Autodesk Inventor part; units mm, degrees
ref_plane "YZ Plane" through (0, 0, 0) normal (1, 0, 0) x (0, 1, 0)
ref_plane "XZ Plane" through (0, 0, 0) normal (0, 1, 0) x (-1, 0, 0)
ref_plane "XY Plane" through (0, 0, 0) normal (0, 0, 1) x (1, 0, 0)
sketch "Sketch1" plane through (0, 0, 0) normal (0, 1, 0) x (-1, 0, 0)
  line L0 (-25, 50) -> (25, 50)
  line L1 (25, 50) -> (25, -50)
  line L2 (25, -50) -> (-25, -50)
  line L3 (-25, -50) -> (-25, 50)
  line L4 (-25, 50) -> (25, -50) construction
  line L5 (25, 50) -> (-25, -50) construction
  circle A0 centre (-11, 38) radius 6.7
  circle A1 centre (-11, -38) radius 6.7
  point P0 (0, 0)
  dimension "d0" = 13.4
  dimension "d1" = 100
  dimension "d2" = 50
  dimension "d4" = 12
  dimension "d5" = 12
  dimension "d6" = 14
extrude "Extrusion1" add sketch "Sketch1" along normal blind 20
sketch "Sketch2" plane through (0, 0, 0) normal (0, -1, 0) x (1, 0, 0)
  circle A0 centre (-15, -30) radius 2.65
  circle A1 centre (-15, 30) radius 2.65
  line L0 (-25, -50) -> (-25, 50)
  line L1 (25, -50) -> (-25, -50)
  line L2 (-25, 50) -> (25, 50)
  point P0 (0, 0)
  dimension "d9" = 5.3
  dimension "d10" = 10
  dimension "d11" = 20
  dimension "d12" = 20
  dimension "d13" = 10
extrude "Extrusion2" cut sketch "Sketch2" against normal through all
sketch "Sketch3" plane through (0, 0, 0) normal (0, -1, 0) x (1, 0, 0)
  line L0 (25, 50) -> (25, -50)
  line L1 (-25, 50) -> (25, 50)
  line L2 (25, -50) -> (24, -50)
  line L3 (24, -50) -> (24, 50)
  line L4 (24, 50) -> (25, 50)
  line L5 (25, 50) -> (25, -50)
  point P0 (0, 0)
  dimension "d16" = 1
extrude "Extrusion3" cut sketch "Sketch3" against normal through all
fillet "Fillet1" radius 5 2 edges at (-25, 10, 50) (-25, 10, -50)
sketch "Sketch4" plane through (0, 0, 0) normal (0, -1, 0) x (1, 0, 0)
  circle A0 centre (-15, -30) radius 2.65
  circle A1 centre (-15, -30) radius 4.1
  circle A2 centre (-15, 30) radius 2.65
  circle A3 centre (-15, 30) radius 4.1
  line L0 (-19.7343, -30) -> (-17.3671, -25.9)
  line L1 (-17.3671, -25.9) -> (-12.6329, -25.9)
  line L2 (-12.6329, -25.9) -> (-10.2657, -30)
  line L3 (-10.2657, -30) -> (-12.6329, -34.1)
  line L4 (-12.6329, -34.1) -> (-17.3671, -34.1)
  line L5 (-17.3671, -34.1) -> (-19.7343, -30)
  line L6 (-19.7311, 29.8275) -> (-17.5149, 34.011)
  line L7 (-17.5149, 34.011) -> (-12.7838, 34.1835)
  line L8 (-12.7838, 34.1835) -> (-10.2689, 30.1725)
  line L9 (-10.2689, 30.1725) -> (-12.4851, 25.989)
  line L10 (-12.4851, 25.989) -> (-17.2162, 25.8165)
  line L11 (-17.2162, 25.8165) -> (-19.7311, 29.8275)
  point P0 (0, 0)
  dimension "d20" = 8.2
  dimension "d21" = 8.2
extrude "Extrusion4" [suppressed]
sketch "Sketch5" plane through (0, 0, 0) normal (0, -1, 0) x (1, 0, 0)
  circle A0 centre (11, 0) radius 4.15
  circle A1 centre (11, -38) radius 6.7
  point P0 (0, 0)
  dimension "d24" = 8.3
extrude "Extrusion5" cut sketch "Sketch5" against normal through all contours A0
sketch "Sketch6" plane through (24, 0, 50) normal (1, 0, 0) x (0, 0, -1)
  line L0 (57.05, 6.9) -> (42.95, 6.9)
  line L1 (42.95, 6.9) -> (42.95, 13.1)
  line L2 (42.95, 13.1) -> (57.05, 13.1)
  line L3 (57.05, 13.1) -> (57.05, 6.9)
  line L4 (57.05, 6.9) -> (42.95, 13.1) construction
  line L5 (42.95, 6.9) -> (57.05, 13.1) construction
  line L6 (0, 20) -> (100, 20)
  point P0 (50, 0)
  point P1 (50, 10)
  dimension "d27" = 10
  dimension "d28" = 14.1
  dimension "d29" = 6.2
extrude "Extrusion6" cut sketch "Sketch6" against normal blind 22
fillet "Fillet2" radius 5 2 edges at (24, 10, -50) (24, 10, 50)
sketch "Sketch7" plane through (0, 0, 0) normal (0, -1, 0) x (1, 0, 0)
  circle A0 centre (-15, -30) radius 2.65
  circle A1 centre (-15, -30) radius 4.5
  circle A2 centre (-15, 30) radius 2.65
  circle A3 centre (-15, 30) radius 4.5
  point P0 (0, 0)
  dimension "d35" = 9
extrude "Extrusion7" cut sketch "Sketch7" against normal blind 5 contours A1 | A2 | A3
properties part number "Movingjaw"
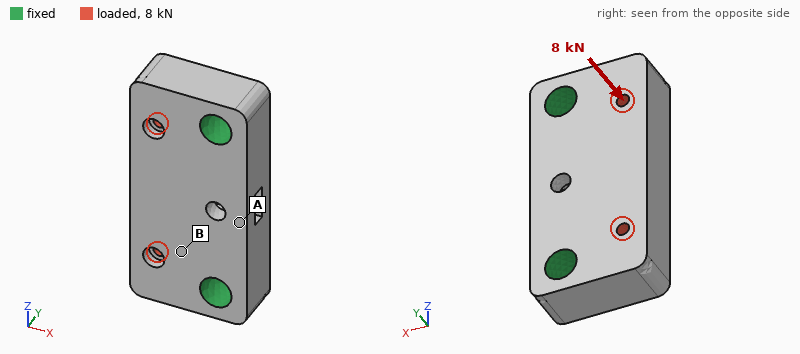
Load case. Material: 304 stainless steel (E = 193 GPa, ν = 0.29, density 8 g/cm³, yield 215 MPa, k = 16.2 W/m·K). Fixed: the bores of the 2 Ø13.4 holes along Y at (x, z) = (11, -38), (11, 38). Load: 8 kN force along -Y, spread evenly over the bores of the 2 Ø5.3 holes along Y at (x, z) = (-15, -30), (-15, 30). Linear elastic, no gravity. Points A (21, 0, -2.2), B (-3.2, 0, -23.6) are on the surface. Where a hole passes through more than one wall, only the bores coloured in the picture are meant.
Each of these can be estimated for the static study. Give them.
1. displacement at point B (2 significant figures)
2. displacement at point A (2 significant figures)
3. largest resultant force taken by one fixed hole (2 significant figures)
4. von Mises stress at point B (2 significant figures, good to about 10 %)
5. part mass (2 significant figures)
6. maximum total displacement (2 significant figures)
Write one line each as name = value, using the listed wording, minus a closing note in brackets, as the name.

displacement at point B = 4.0 µm
displacement at point A = 1.9 µm
largest resultant force taken by one fixed hole = 4.0 kN
von Mises stress at point B = 13 MPa
part mass = 700 g
maximum total displacement = 10 µm
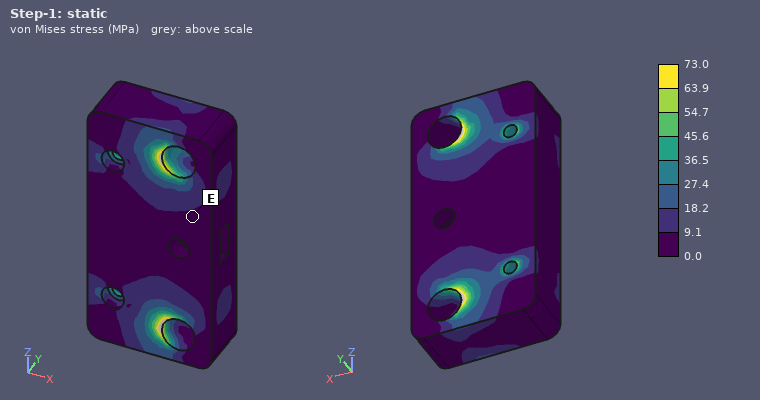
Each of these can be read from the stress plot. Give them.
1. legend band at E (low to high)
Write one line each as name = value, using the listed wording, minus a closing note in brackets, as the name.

legend band at E = 0.0 to 9.1 MPa
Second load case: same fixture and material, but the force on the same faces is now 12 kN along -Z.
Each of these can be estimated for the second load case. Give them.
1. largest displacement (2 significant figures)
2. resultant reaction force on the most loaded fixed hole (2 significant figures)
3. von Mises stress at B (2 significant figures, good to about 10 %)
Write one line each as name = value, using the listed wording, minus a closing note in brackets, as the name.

largest displacement = 4.1 µm
resultant reaction force on the most loaded fixed hole = 6.8 kN
von Mises stress at B = 11 MPa
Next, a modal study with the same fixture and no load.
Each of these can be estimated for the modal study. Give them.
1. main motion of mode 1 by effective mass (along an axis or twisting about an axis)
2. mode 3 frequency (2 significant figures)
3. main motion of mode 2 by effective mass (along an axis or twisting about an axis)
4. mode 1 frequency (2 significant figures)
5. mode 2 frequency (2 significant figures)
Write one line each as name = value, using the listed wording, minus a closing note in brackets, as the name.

main motion of mode 1 by effective mass = along Y
mode 3 frequency = 16 kHz
main motion of mode 2 by effective mass = twisting about X
mode 1 frequency = 8600 Hz
mode 2 frequency = 14 kHz
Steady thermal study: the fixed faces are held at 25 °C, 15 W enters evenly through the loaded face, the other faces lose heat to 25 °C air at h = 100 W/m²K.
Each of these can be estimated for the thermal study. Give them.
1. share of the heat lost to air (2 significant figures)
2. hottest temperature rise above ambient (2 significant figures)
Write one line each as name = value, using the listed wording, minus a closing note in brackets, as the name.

share of the heat lost to air = 44 %
hottest temperature rise above ambient = 16 K
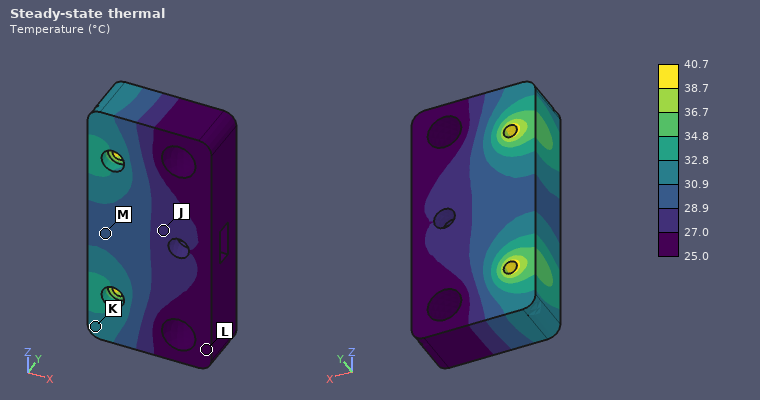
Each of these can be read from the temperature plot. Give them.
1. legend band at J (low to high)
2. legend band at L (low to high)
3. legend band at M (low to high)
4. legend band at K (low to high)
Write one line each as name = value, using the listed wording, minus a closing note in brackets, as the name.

legend band at J = 27.0 to 28.9 °C
legend band at L = 25.0 to 27.0 °C
legend band at M = 28.9 to 30.9 °C
legend band at K = 30.9 to 32.8 °C
